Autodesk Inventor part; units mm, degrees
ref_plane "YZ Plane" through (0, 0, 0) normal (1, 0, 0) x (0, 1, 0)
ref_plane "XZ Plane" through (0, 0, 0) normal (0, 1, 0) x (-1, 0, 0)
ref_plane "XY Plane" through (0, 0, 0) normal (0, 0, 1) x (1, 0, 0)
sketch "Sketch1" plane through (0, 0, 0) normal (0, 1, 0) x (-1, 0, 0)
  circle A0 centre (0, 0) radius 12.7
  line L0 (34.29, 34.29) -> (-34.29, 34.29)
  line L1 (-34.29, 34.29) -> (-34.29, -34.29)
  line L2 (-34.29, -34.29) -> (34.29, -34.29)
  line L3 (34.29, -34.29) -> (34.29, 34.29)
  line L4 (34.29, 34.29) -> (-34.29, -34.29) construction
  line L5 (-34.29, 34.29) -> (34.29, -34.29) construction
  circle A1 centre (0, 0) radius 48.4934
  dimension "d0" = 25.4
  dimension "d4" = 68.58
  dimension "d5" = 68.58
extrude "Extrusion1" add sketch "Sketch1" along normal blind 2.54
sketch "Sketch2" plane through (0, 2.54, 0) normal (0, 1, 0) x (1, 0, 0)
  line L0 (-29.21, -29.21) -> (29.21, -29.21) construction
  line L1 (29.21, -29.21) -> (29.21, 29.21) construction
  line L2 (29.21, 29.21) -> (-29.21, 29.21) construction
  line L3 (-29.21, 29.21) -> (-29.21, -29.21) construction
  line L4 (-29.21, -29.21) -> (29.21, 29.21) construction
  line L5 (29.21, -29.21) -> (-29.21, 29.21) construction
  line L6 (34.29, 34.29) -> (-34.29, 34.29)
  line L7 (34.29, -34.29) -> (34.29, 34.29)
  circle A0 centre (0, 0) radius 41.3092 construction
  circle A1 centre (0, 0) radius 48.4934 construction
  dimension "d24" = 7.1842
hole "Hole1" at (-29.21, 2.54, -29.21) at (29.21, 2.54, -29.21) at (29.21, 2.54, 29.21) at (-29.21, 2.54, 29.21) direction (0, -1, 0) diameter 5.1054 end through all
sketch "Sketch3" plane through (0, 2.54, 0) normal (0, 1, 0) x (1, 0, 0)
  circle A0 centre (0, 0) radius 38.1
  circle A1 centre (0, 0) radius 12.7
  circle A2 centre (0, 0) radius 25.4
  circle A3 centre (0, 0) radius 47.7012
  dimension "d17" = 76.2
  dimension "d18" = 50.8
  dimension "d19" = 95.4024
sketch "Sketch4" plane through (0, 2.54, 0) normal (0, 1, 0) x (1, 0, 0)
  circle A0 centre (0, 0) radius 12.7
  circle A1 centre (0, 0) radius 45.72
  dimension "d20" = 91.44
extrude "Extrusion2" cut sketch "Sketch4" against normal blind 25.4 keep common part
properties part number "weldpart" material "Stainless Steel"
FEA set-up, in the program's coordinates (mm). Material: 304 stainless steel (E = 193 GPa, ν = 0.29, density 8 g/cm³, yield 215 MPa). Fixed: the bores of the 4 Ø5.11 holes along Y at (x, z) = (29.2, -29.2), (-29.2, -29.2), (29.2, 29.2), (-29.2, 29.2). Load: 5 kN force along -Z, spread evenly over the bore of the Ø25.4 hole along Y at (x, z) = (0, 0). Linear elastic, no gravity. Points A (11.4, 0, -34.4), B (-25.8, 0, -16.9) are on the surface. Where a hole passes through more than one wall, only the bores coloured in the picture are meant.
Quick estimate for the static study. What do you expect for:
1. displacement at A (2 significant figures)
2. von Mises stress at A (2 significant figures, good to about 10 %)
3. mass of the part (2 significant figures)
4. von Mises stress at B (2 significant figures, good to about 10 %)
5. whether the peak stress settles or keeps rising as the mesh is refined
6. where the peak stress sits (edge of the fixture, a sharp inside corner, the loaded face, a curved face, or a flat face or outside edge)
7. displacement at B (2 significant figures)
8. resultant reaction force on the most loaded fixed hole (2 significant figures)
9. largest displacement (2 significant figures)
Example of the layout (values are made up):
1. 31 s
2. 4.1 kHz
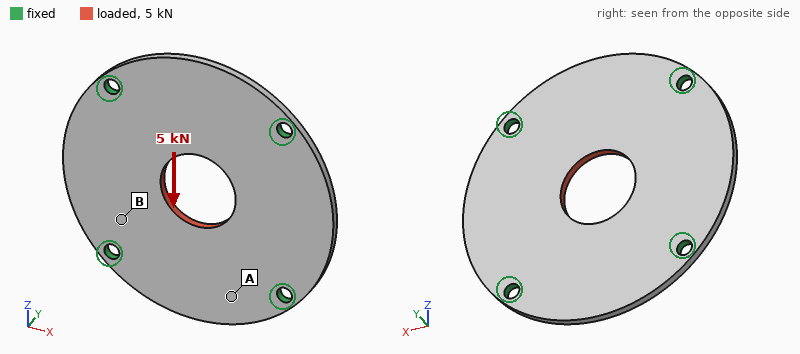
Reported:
1. 3.7 µm
2. 11 MPa
3. 120 g
4. 23 MPa
5. keeps rising
6. edge of the fixture
7. 1.7 µm
8. 1.3 kN
9. 5.9 µm
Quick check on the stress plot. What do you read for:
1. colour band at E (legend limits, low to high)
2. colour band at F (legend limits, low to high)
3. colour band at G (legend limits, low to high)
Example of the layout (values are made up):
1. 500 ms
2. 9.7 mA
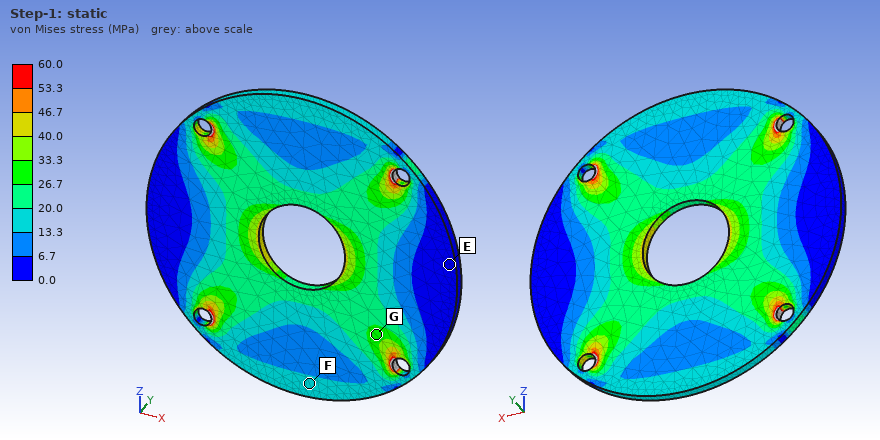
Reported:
1. 0.0 to 6.7 MPa
2. 13.3 to 20.0 MPa
3. 26.7 to 33.3 MPa
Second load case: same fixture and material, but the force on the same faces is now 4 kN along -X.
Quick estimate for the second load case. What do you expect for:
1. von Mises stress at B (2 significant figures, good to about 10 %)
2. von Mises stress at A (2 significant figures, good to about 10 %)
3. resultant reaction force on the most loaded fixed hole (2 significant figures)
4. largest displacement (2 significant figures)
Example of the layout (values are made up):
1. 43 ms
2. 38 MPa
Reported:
1. 17 MPa
2. 5.7 MPa
3. 1.0 kN
4. 4.8 µm
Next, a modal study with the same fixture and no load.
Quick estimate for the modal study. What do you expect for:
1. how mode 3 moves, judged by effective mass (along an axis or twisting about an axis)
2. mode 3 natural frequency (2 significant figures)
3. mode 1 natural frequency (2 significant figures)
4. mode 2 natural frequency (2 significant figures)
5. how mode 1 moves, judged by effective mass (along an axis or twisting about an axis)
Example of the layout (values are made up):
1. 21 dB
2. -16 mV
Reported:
1. twisting about X
2. 3500 Hz
3. 3000 Hz
4. 3300 Hz
5. along Y
